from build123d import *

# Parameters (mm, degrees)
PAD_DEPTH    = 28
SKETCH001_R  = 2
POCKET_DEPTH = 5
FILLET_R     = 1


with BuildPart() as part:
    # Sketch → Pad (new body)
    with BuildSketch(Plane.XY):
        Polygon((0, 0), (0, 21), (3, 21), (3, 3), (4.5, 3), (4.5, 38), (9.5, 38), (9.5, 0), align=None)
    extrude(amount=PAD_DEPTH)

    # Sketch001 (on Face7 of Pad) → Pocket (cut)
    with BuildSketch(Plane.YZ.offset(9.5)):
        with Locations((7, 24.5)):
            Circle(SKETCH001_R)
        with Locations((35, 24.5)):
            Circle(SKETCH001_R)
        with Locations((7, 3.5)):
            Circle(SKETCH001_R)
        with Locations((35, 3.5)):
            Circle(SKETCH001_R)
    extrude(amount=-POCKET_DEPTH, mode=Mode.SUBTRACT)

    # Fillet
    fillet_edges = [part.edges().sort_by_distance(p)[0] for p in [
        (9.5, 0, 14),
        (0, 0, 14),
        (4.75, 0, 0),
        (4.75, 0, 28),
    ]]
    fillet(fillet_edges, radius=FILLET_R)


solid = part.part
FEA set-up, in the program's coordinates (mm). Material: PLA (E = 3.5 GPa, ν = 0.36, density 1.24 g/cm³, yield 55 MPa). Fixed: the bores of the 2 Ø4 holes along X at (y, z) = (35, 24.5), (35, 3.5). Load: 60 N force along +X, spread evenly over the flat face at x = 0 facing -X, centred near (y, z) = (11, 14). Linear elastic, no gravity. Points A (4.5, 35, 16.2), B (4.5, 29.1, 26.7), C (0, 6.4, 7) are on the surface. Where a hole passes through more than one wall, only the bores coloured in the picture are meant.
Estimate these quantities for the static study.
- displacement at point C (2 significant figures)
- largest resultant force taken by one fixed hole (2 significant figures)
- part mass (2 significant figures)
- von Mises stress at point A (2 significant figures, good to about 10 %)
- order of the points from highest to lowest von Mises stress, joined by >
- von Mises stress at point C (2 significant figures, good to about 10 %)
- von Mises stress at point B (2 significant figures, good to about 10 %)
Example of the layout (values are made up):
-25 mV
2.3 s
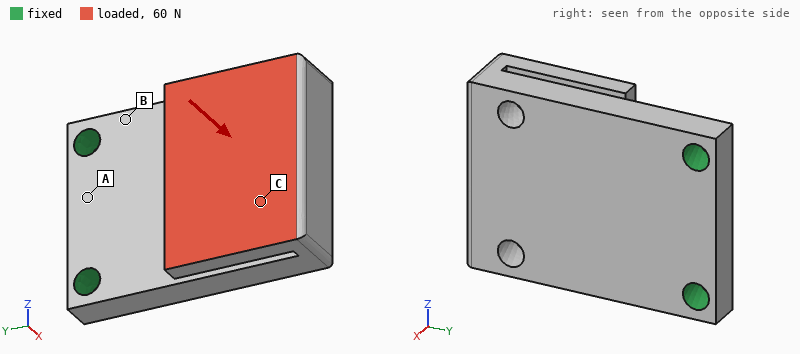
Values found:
0.44 mm
30 N
8.6 g
2.9 MPa
B > C > A
6.9 MPa
11 MPa
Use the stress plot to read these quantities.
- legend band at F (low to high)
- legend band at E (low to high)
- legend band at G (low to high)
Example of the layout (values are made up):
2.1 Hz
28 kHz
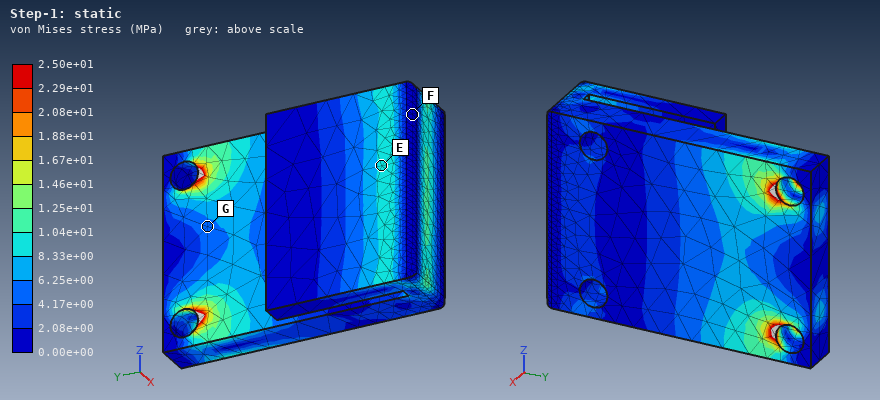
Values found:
0.00e+00 to 2.08e+00 MPa
8.33e+00 to 1.04e+01 MPa
4.17e+00 to 6.25e+00 MPa
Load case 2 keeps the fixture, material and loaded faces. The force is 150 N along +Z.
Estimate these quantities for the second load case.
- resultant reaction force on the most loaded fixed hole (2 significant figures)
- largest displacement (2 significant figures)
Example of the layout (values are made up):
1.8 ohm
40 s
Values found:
180 N
0.45 mm
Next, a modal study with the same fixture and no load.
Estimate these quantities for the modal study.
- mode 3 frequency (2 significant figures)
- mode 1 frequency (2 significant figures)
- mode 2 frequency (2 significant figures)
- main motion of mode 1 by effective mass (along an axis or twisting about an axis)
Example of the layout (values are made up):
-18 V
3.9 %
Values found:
1800 Hz
820 Hz
1600 Hz
along X
